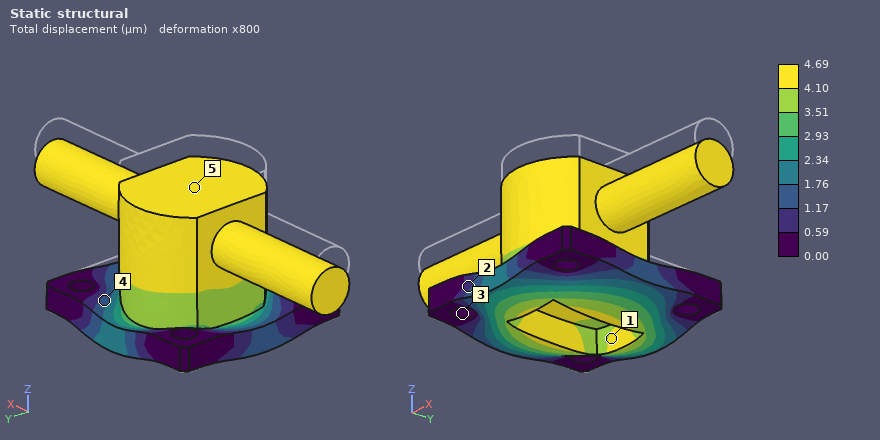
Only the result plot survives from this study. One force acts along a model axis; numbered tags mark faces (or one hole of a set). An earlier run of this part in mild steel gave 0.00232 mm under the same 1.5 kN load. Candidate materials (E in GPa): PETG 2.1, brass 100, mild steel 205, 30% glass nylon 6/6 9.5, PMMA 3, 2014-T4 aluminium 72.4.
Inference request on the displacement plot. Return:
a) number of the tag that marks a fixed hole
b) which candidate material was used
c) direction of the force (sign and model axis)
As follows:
3
brass
-Z
